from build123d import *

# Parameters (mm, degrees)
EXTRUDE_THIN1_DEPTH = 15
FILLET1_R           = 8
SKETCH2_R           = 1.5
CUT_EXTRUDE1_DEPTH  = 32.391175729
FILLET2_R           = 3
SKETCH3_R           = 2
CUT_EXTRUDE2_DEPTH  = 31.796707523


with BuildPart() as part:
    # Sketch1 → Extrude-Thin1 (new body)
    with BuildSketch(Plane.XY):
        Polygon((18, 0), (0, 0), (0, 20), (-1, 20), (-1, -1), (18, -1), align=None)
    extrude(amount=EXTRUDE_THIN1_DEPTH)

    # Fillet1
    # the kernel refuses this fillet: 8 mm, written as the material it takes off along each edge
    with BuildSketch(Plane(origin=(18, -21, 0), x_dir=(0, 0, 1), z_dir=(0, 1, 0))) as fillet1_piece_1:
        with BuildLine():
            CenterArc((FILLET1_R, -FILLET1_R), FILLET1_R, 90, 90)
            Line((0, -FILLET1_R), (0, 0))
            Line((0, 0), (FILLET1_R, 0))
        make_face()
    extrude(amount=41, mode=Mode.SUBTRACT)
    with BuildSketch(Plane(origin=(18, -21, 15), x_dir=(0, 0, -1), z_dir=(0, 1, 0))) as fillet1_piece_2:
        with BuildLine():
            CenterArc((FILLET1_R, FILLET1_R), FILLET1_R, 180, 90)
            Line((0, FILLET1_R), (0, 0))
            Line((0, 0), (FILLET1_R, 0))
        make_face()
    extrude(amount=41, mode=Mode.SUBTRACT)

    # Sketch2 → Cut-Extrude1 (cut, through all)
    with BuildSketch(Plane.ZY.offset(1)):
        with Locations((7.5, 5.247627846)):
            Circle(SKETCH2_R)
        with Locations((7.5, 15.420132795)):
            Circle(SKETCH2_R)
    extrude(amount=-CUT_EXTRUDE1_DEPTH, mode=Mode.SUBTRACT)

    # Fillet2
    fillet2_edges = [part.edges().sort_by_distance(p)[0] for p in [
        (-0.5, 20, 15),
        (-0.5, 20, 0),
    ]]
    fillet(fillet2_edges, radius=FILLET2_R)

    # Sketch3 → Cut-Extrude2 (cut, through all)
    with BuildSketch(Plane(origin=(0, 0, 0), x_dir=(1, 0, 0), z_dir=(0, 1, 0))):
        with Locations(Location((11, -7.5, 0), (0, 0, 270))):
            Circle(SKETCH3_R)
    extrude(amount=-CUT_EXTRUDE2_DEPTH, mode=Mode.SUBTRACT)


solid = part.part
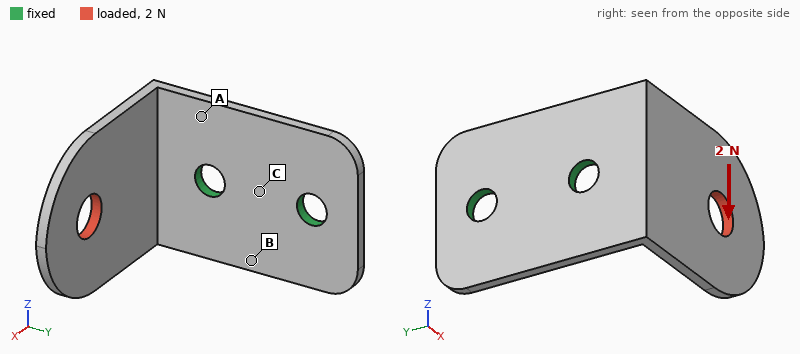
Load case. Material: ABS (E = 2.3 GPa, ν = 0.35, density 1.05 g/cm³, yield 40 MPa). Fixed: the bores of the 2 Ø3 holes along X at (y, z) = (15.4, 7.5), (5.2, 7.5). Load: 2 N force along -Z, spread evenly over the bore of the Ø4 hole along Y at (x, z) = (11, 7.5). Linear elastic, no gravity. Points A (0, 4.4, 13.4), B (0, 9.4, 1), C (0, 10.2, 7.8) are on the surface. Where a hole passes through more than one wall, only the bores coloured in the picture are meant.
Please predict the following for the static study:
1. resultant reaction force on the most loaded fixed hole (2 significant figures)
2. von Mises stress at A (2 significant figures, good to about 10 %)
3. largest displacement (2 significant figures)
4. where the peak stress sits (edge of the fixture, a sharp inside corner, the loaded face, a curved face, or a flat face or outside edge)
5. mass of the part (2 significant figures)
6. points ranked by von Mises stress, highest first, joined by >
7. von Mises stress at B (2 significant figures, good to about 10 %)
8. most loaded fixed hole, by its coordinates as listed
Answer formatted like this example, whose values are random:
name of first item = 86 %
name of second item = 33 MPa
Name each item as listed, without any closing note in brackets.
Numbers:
resultant reaction force on the most loaded fixed hole = 2.7 N
von Mises stress at A = 3.4 MPa
largest displacement = 0.36 mm
where the peak stress sits = a flat face or outside edge
mass of the part = 0.55 g
points ranked by von Mises stress, highest first, joined by > = A > B > C
von Mises stress at B = 1.8 MPa
most loaded fixed hole, by its coordinates as listed = (5.2, 7.5)
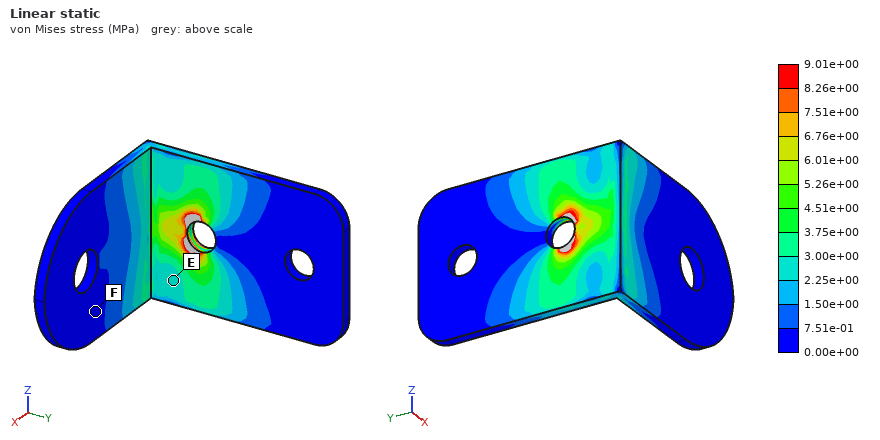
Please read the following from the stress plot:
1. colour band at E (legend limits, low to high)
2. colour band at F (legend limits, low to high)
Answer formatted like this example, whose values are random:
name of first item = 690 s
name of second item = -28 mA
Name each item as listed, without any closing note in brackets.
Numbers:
colour band at E = 2.25e+00 to 3.00e+00 MPa
colour band at F = 0.00e+00 to 7.51e-01 MPa
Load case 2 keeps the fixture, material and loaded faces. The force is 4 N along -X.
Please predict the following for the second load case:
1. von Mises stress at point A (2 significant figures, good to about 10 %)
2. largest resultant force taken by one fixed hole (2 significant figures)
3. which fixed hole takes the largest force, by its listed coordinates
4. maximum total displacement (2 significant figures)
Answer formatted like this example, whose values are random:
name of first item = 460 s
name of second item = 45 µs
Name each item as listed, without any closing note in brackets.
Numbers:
von Mises stress at point A = 2.8 MPa
largest resultant force taken by one fixed hole = 4.3 N
which fixed hole takes the largest force, by its listed coordinates = (5.2, 7.5)
maximum total displacement = 0.35 mm
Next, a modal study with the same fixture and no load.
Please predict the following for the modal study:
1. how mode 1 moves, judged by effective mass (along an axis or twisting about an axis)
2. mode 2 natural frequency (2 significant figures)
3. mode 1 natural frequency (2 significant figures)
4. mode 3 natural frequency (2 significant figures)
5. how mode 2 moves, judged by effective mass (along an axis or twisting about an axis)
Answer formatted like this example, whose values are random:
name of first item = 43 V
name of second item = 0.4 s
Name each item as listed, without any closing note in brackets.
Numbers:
how mode 1 moves, judged by effective mass = along Y
mode 2 natural frequency = 1000 Hz
mode 1 natural frequency = 600 Hz
mode 3 natural frequency = 2300 Hz
how mode 2 moves, judged by effective mass = along Z
